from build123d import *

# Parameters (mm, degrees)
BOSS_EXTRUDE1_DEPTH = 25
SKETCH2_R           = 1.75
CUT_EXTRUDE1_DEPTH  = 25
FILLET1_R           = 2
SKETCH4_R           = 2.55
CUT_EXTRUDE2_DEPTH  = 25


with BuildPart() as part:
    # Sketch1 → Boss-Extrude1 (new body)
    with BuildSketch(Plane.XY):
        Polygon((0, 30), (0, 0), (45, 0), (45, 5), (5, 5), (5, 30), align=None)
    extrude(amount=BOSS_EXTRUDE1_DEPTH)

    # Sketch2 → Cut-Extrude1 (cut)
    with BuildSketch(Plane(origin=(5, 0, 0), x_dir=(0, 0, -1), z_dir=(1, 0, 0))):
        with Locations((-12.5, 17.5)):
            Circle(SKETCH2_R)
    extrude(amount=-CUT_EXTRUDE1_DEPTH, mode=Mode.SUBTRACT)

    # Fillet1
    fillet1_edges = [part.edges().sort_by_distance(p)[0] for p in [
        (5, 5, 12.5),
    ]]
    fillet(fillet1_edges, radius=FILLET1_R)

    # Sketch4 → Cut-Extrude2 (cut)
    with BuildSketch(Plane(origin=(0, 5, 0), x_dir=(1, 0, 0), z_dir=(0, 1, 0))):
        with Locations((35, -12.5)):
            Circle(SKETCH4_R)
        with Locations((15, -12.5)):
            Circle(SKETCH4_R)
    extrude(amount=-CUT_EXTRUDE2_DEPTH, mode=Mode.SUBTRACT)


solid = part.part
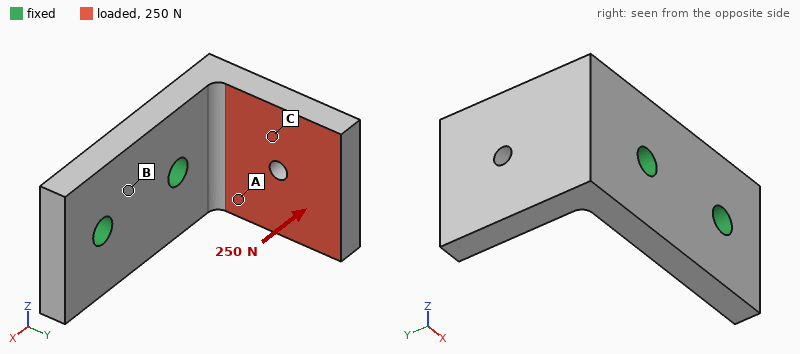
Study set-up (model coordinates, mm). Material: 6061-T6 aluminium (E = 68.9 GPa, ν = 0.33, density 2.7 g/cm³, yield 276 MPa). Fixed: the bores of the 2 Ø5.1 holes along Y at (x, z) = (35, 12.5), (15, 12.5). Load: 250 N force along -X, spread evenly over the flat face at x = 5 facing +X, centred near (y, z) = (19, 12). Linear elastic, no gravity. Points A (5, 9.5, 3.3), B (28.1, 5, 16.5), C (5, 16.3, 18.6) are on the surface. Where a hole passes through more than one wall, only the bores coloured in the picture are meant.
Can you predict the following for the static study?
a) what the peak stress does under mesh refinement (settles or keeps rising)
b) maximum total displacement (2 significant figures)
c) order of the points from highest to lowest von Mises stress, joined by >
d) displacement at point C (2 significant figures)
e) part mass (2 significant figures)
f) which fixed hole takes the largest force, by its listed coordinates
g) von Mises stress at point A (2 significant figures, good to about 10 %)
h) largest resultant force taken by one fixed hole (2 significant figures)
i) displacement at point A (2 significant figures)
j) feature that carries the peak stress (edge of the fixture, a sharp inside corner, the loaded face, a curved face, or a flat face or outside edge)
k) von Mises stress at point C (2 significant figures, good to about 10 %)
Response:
keeps rising
0.10 mm
A > C > B
0.044 mm
23 g
(15, 12.5)
21 MPa
220 N
0.021 mm
edge of the fixture
11 MPa
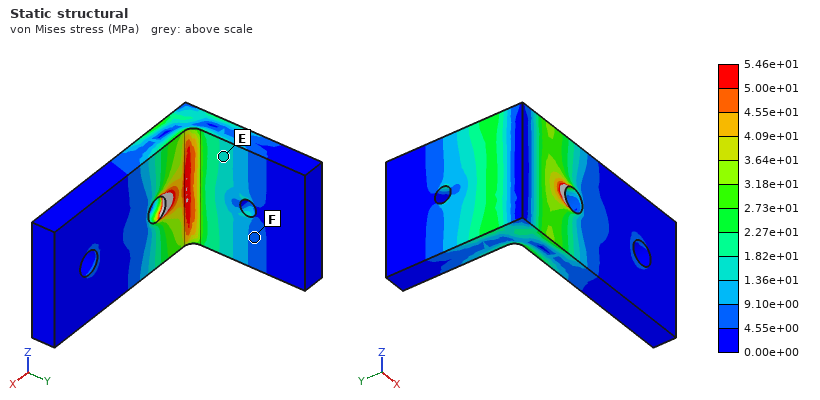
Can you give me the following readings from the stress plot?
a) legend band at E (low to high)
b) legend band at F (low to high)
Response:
1.36e+01 to 1.82e+01 MPa
4.55e+00 to 9.10e+00 MPa
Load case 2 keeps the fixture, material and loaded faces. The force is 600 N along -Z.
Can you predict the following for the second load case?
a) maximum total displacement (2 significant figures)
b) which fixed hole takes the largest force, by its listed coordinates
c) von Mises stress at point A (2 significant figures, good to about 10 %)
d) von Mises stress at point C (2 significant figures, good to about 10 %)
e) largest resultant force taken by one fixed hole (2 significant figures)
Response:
0.12 mm
(15, 12.5)
34 MPa
21 MPa
790 N
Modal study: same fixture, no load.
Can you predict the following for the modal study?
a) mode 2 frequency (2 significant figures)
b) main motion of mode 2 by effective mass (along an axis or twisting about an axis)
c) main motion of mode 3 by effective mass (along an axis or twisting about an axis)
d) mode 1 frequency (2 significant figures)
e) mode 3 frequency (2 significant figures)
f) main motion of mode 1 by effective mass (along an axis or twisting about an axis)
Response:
4700 Hz
along Z
along Y
3400 Hz
11 kHz
along X
